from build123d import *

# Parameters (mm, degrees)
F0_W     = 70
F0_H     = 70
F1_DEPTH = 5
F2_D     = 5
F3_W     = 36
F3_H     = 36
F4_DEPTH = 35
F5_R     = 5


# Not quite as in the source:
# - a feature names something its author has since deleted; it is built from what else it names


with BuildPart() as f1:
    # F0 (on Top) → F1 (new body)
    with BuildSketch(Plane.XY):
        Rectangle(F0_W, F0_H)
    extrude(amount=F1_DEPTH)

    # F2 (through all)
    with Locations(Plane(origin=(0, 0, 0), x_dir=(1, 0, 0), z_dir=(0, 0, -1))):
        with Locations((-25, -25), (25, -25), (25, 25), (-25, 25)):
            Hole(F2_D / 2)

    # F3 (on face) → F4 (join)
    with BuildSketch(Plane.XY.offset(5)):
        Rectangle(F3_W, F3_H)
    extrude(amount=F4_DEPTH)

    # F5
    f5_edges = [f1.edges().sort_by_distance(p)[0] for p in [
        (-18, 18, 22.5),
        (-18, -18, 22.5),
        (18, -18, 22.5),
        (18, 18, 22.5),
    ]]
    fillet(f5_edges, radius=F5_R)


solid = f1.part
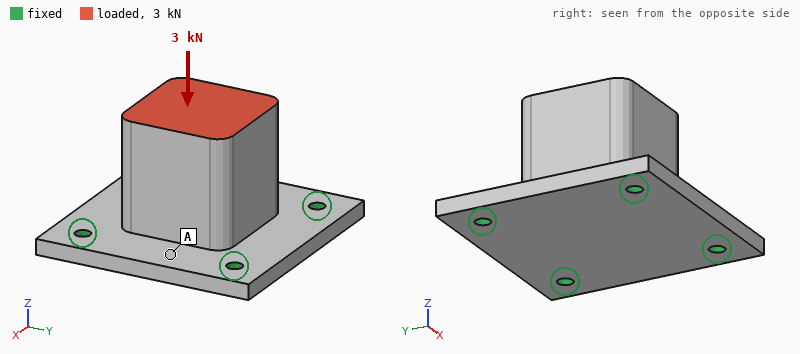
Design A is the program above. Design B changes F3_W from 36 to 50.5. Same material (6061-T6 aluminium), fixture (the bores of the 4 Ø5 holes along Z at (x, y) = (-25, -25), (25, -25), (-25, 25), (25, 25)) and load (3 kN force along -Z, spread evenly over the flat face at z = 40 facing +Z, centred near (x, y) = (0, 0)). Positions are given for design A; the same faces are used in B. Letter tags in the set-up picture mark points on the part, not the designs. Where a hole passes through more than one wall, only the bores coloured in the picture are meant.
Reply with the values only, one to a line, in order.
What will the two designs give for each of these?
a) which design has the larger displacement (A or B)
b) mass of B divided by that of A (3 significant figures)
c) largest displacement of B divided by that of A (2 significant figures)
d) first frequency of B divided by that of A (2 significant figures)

A
1.27
0.54
1.2
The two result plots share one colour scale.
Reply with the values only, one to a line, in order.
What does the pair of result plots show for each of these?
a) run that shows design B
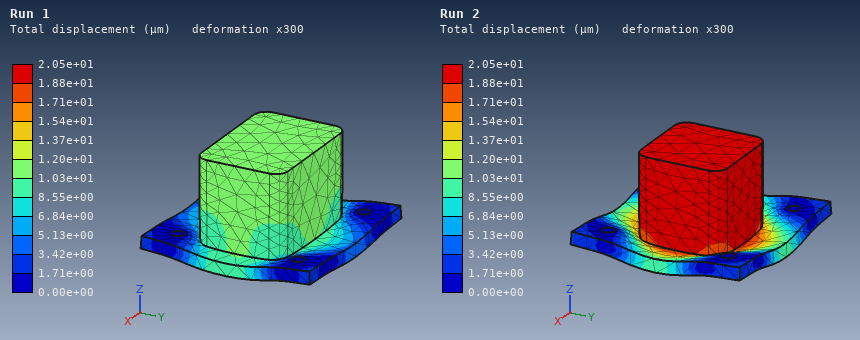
Run 1
